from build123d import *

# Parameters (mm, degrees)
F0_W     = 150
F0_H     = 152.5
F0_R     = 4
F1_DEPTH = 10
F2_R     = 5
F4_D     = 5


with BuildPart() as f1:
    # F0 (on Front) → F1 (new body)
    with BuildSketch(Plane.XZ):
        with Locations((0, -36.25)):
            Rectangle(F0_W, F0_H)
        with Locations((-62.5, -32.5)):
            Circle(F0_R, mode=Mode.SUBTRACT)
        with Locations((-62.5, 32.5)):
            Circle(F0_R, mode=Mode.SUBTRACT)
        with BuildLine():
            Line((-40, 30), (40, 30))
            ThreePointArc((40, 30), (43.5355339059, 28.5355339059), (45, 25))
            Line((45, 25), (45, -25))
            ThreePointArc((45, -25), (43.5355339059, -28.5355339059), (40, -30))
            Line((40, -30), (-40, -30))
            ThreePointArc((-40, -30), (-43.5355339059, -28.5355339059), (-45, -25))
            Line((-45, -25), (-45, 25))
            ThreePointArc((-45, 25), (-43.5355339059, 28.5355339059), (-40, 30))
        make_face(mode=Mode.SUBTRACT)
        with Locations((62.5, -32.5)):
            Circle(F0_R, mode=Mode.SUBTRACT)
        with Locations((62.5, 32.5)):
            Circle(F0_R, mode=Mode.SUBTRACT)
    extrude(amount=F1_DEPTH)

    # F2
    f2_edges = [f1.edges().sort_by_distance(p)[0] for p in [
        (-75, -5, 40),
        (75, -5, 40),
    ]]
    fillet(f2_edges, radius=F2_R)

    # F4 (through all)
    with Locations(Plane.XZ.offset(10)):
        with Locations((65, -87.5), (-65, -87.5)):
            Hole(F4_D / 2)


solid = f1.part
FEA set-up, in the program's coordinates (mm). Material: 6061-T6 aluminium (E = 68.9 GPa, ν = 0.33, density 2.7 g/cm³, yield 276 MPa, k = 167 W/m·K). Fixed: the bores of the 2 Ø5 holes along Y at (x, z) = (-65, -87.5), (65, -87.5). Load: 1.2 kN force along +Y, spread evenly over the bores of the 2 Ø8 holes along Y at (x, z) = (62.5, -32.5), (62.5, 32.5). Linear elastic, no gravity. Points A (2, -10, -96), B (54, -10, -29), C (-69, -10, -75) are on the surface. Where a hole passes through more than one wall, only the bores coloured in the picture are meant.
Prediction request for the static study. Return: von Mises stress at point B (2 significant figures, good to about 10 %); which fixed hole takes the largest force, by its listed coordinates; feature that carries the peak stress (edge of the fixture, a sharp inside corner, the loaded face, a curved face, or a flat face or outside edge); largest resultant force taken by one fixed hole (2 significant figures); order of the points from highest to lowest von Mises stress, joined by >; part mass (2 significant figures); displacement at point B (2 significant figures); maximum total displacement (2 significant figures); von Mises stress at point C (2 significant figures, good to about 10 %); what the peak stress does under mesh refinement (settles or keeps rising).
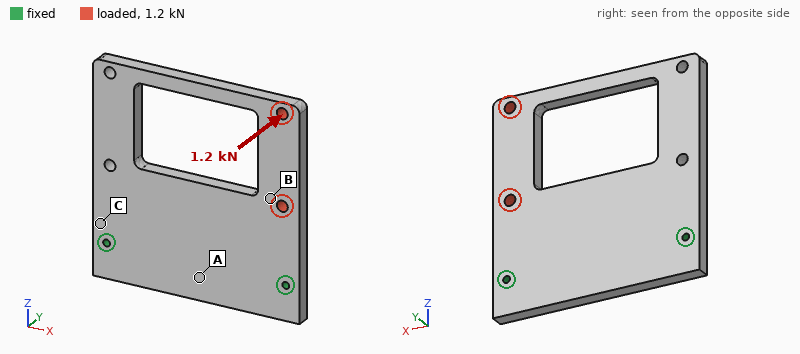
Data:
66 MPa
(65, -87.5)
edge of the fixture
1.2 kN
B > C > A
470 g
0.46 mm
1.6 mm
43 MPa
keeps rising
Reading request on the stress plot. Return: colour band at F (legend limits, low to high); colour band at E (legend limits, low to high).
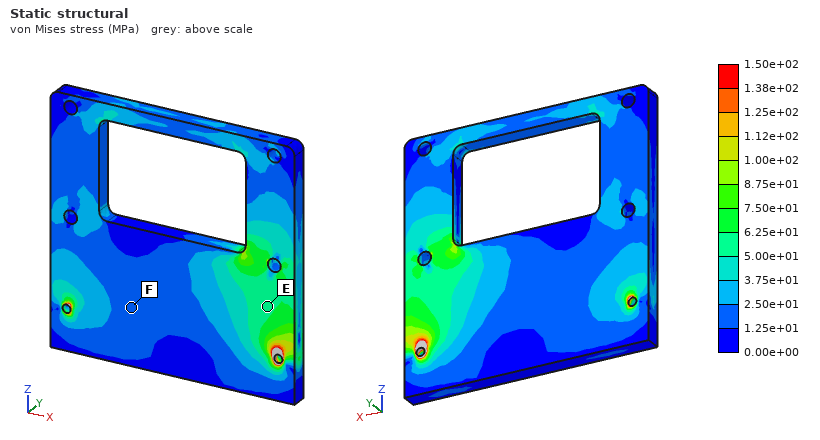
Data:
1.25e+01 to 2.50e+01 MPa
5.00e+01 to 6.25e+01 MPa
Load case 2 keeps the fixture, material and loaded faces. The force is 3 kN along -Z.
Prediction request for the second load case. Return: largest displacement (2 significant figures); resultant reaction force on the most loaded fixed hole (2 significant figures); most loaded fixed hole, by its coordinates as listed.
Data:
22 µm
2.9 kN
(65, -87.5)
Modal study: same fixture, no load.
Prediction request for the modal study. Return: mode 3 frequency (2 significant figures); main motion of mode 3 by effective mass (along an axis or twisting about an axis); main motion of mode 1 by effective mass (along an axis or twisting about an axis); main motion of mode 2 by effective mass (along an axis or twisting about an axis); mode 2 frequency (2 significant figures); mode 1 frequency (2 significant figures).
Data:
1900 Hz
along Y
along Y
twisting about Z
880 Hz
460 Hz
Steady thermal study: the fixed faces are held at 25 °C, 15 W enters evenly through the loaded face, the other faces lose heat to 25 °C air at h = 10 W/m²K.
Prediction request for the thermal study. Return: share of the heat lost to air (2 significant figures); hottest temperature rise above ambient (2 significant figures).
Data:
13 %
17 K
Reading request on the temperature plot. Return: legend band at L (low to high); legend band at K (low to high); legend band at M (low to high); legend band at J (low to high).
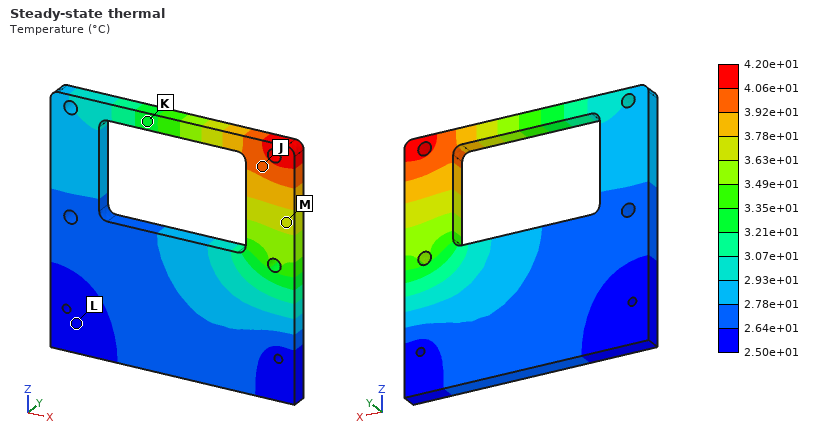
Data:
2.50e+01 to 2.64e+01 °C
3.21e+01 to 3.35e+01 °C
3.63e+01 to 3.78e+01 °C
3.92e+01 to 4.06e+01 °C
